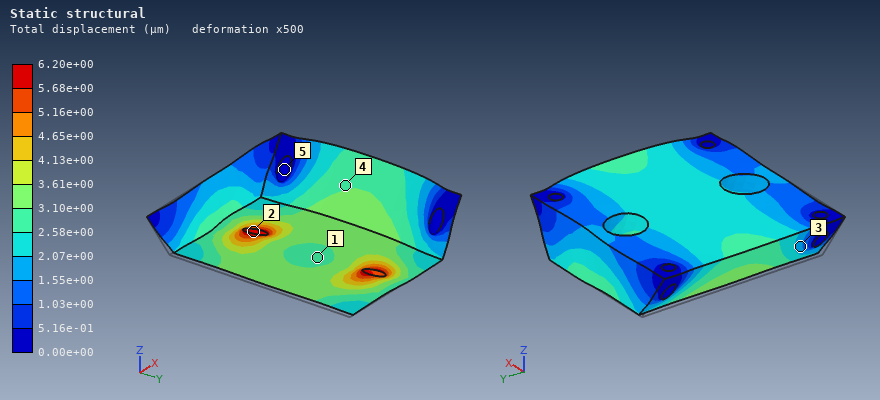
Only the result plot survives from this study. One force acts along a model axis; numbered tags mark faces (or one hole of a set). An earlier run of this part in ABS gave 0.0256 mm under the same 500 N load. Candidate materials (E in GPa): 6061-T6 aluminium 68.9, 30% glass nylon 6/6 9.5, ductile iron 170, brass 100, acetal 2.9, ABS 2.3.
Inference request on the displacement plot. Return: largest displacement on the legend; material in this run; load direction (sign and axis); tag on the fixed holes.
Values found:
6.20e+00 µm
30% glass nylon 6/6
+X
5
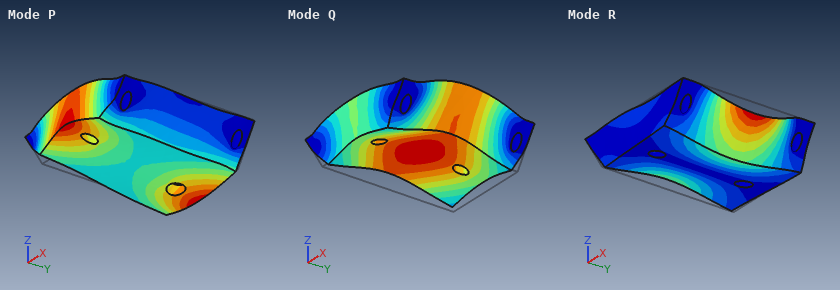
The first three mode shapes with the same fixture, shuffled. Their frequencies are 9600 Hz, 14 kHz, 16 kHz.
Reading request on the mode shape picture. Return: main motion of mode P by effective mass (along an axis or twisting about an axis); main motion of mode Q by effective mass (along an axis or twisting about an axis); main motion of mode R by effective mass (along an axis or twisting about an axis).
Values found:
along Y
along Z
along X
